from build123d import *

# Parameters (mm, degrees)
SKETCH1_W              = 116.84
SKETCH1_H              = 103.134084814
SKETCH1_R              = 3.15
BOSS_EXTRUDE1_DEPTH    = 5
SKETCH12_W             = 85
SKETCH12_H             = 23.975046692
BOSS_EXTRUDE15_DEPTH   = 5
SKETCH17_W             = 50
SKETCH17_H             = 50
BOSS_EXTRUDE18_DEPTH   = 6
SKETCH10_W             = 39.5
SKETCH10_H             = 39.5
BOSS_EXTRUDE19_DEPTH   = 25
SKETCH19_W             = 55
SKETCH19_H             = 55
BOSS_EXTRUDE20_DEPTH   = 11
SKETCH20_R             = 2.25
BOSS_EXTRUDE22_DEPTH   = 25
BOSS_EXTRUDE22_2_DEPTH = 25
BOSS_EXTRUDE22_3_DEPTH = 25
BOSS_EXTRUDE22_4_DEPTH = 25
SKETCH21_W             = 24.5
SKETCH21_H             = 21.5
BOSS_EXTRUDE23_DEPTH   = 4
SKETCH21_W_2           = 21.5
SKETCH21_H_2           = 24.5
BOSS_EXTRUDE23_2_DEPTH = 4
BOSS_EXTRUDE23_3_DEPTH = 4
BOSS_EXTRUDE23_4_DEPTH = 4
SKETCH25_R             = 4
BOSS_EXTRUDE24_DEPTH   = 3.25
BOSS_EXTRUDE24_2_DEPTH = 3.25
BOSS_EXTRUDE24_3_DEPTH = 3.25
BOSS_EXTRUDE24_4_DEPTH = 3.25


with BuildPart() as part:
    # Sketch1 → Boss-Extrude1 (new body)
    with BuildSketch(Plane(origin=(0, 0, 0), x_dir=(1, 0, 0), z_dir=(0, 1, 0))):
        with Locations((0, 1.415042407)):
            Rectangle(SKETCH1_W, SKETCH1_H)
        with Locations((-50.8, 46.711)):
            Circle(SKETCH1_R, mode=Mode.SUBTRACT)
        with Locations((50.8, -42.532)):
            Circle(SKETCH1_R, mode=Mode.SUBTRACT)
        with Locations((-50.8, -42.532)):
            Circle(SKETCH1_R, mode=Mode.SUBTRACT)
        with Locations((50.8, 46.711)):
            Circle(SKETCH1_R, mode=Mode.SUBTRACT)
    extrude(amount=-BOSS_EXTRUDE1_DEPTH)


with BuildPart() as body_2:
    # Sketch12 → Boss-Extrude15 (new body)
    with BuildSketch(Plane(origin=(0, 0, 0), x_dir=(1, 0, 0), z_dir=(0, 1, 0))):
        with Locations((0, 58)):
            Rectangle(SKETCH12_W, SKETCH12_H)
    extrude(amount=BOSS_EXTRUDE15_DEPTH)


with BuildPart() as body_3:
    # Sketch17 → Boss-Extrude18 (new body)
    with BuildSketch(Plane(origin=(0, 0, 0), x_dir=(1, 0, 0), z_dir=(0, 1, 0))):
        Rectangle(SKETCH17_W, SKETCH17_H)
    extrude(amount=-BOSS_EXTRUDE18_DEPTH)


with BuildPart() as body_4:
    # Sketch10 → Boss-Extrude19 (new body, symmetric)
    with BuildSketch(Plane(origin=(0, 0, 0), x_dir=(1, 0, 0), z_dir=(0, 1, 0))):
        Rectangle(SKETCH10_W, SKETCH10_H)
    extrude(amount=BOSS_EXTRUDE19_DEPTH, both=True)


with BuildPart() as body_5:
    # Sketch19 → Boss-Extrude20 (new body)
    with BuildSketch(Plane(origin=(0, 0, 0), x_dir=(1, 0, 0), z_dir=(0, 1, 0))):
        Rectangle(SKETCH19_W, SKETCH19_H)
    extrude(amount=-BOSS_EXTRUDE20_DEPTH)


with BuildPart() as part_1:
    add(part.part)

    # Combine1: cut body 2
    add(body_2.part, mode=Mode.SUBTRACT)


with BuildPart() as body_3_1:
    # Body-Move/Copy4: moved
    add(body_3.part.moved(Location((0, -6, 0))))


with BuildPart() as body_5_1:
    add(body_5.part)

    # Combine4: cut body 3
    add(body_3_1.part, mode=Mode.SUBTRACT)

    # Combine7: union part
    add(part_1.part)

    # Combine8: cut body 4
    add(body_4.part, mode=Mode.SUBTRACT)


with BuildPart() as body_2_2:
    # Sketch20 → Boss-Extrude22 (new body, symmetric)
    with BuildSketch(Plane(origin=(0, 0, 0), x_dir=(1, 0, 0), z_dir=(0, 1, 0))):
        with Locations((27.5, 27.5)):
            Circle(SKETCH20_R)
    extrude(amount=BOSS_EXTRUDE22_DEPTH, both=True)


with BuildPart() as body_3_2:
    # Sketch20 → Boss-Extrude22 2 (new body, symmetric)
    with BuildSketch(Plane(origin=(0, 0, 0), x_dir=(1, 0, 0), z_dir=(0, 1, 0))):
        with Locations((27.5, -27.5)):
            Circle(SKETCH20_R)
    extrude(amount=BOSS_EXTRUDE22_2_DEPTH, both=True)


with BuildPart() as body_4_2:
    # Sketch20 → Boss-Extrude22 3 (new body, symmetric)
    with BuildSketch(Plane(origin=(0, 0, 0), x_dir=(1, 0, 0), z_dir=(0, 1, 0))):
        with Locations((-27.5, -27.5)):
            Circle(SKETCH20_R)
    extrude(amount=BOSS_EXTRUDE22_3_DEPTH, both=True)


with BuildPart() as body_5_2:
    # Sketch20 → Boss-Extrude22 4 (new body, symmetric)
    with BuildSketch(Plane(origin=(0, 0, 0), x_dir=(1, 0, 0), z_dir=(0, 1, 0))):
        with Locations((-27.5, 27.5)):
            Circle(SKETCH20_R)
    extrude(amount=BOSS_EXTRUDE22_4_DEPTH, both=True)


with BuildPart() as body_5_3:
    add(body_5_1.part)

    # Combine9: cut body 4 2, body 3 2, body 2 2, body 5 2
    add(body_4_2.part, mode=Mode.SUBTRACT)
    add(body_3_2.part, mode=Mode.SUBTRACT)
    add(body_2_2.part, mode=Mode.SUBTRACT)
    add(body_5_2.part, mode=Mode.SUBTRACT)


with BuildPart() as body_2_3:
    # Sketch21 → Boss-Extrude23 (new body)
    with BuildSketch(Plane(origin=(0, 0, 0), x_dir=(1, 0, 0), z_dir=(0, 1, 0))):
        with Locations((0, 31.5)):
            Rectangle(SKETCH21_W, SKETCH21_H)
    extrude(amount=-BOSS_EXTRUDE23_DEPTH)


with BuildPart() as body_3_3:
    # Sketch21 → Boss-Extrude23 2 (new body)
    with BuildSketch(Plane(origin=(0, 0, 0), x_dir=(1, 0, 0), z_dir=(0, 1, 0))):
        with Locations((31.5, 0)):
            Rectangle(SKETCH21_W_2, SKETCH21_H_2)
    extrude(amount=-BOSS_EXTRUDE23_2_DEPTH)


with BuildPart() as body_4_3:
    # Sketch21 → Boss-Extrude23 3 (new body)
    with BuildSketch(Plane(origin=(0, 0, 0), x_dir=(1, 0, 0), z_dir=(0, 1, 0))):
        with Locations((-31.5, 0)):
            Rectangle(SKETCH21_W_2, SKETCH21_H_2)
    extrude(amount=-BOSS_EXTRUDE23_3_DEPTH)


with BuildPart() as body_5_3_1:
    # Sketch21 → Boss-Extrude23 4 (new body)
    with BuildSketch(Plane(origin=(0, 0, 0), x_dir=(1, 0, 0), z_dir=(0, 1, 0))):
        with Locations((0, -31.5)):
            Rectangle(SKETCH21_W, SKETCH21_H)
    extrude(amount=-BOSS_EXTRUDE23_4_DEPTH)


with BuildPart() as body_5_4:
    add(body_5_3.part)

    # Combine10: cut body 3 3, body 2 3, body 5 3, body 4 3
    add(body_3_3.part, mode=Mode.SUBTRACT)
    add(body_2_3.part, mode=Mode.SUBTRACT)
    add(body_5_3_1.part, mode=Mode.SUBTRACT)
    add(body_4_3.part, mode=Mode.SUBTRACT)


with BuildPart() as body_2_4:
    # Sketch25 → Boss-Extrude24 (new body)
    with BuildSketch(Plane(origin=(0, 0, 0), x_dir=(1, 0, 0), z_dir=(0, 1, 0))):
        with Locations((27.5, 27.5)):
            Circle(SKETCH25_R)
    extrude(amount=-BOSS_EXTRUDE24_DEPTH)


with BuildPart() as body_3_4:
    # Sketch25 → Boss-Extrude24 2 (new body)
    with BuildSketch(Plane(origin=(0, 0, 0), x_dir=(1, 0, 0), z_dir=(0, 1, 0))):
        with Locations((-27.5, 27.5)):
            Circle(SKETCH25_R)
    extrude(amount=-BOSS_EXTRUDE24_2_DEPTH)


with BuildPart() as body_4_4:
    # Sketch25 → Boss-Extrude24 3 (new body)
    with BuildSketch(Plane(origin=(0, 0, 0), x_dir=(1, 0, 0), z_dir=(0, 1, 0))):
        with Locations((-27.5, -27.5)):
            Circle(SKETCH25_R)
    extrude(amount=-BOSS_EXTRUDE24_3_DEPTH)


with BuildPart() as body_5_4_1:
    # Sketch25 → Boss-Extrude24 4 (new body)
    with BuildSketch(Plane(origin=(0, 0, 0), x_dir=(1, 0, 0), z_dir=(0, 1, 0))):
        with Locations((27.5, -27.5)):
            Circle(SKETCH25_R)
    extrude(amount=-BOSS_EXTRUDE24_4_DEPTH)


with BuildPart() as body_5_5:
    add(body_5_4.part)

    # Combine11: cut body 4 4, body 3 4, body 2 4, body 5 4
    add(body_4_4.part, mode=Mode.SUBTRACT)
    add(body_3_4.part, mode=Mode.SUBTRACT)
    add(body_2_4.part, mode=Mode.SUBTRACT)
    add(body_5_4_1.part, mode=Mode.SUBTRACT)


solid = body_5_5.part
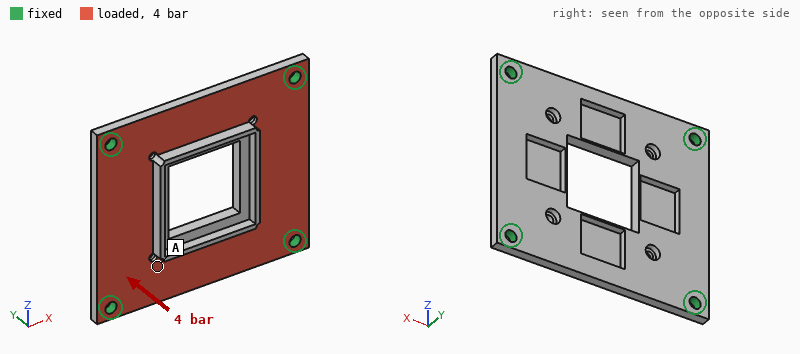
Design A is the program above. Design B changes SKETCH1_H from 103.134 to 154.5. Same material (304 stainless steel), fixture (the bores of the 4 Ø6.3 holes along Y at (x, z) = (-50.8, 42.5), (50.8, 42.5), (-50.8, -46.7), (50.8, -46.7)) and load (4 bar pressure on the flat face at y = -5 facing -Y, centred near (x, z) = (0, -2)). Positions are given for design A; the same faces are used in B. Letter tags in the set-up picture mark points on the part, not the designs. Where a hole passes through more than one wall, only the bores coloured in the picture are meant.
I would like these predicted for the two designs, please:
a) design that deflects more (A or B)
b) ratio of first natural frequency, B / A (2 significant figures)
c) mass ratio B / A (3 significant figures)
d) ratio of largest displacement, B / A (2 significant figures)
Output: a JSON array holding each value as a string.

["B", "0.85", "1.64", "1.8"]
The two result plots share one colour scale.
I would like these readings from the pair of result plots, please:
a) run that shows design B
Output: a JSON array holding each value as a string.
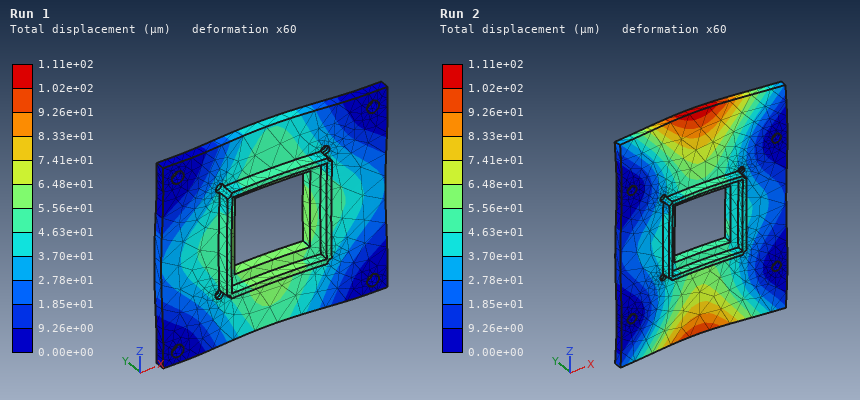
["Run 2"]
